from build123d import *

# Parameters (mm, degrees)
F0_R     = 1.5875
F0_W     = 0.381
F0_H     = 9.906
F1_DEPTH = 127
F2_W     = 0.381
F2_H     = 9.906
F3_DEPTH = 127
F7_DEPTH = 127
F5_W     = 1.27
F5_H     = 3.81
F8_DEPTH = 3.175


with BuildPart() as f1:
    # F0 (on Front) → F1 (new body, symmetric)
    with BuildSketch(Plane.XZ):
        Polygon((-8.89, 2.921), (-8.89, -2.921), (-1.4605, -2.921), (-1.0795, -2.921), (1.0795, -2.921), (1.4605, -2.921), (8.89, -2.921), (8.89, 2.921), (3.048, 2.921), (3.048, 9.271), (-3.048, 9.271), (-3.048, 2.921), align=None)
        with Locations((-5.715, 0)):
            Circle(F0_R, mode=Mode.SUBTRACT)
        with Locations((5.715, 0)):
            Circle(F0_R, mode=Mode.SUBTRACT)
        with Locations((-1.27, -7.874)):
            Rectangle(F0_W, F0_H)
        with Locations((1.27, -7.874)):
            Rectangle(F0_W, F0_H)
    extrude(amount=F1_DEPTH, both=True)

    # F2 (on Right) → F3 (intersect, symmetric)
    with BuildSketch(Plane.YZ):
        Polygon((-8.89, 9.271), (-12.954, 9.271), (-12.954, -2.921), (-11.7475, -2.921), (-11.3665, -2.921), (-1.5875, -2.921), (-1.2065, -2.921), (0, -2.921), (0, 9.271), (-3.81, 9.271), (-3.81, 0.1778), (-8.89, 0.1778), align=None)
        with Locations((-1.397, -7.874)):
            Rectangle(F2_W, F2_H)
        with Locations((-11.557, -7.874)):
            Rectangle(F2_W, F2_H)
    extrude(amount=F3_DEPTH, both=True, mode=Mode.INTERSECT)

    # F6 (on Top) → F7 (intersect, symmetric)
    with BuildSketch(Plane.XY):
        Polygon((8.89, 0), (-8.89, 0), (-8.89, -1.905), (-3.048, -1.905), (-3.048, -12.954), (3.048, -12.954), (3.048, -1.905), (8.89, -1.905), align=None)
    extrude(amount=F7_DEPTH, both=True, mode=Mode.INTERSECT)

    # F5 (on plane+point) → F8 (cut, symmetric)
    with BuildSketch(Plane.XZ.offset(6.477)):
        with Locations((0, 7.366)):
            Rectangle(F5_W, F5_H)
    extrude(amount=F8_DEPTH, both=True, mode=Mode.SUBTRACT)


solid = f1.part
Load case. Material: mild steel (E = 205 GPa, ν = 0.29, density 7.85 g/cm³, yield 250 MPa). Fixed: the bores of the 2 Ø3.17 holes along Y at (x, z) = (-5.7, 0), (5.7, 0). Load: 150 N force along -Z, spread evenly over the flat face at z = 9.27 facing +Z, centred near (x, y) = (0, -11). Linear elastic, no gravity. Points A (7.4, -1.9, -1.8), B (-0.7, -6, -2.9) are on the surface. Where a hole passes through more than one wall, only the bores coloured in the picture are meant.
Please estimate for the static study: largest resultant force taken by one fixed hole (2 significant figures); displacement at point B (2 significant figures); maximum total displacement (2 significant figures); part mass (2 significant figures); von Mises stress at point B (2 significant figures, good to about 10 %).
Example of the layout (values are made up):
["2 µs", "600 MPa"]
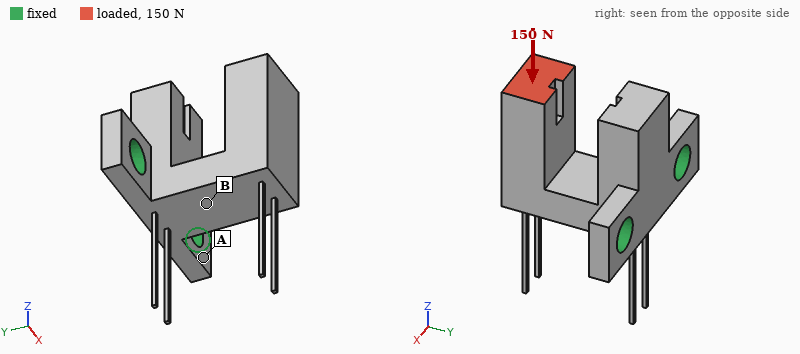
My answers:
["80 N", "10 µm", "44 µm", "6.1 g", "74 MPa"]
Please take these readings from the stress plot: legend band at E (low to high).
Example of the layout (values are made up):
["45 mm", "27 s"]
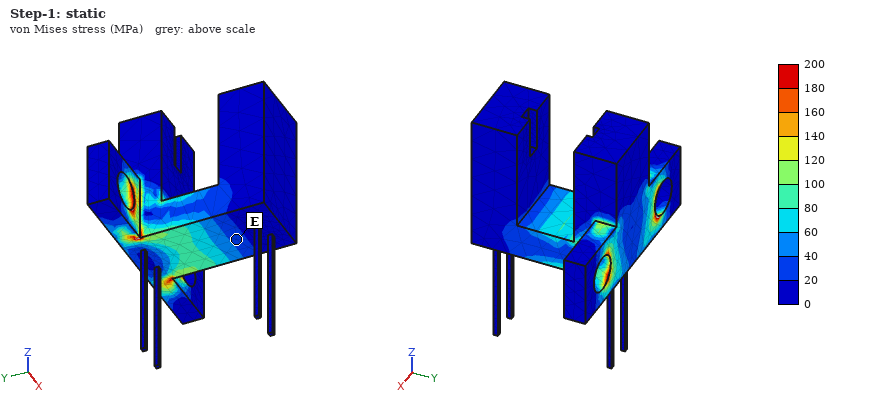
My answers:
["20 to 40 MPa"]
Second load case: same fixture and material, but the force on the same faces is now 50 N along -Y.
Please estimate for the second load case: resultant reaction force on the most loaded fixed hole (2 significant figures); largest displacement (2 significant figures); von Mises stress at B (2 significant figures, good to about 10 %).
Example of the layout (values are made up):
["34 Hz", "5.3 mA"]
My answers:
["25 N", "24 µm", "51 MPa"]
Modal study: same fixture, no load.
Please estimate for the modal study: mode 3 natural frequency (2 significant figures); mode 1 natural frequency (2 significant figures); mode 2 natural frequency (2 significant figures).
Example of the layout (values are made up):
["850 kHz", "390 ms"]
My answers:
["3100 Hz", "3100 Hz", "3100 Hz"]
